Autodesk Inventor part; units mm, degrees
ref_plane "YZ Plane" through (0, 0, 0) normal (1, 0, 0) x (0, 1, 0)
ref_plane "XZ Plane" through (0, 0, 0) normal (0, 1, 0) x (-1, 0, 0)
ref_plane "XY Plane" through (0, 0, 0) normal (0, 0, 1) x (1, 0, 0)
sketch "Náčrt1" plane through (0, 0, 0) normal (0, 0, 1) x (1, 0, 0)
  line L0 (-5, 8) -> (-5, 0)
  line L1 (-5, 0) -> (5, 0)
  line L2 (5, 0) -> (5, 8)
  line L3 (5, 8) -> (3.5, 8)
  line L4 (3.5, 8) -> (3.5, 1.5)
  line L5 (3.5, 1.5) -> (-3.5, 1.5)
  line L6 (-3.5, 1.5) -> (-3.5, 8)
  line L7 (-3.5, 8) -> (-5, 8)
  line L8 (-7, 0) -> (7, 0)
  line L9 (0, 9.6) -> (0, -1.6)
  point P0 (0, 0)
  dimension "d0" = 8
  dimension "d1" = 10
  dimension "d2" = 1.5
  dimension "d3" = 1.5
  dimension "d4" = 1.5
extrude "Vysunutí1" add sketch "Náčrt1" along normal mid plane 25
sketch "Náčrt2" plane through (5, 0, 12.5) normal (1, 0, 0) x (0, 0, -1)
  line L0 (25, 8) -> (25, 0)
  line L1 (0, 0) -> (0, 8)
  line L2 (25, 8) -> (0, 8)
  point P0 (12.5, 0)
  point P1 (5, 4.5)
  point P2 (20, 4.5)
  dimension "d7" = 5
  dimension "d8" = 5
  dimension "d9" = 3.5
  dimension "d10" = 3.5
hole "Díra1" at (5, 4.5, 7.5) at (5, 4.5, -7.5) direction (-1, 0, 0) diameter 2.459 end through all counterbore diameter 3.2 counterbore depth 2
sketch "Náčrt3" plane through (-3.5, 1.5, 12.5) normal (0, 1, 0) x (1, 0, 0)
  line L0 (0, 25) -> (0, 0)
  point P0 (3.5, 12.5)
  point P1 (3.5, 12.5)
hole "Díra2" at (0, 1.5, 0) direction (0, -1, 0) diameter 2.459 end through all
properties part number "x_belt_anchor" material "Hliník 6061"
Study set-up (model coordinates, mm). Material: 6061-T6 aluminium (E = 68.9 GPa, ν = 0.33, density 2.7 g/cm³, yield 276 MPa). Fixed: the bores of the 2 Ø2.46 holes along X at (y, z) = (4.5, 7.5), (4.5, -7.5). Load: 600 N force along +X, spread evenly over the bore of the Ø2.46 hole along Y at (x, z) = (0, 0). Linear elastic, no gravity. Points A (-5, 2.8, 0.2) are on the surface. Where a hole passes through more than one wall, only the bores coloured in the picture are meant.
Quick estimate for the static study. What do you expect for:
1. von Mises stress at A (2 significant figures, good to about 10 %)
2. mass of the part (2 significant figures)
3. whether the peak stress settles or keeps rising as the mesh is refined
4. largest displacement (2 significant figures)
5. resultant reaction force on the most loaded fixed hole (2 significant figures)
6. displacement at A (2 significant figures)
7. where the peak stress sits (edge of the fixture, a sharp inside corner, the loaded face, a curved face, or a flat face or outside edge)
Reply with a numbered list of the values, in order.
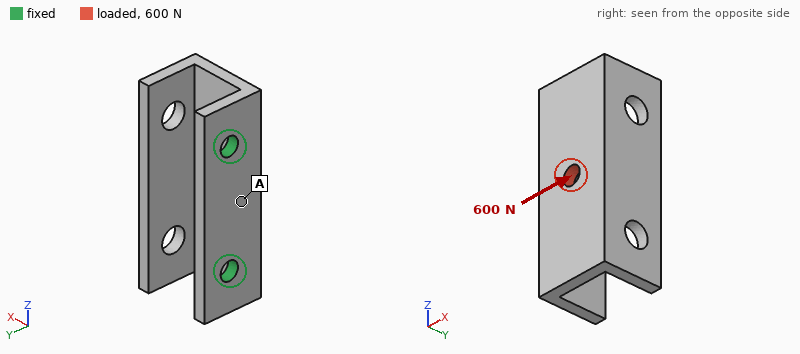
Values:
1. 51 MPa
2. 2.2 g
3. keeps rising
4. 87 µm
5. 310 N
6. 15 µm
7. edge of the fixture
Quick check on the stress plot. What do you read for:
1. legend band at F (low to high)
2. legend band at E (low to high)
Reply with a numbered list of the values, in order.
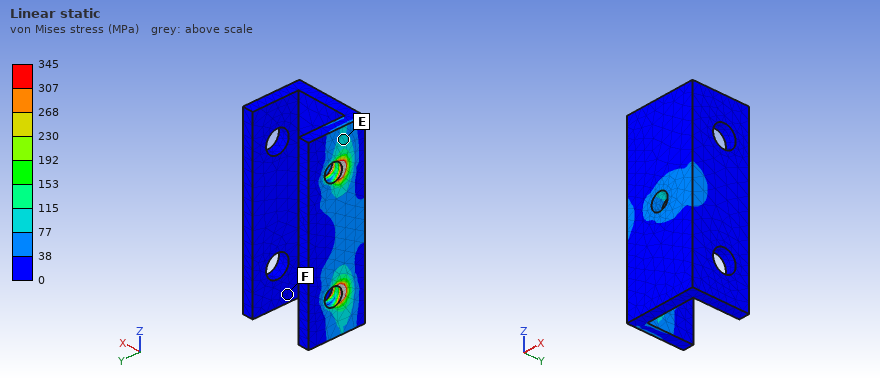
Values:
1. 0 to 38 MPa
2. 77 to 115 MPa
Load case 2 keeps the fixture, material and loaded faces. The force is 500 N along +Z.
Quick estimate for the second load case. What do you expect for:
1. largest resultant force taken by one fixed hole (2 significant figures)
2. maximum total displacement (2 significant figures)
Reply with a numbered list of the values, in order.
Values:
1. 300 N
2. 29 µm
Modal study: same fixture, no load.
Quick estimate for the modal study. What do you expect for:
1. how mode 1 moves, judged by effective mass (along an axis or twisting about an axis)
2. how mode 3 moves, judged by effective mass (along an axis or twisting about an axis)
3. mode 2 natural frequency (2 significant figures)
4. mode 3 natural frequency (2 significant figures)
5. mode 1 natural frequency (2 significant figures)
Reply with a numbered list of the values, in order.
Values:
1. along Y
2. along X
3. 8400 Hz
4. 14 kHz
5. 5100 Hz
